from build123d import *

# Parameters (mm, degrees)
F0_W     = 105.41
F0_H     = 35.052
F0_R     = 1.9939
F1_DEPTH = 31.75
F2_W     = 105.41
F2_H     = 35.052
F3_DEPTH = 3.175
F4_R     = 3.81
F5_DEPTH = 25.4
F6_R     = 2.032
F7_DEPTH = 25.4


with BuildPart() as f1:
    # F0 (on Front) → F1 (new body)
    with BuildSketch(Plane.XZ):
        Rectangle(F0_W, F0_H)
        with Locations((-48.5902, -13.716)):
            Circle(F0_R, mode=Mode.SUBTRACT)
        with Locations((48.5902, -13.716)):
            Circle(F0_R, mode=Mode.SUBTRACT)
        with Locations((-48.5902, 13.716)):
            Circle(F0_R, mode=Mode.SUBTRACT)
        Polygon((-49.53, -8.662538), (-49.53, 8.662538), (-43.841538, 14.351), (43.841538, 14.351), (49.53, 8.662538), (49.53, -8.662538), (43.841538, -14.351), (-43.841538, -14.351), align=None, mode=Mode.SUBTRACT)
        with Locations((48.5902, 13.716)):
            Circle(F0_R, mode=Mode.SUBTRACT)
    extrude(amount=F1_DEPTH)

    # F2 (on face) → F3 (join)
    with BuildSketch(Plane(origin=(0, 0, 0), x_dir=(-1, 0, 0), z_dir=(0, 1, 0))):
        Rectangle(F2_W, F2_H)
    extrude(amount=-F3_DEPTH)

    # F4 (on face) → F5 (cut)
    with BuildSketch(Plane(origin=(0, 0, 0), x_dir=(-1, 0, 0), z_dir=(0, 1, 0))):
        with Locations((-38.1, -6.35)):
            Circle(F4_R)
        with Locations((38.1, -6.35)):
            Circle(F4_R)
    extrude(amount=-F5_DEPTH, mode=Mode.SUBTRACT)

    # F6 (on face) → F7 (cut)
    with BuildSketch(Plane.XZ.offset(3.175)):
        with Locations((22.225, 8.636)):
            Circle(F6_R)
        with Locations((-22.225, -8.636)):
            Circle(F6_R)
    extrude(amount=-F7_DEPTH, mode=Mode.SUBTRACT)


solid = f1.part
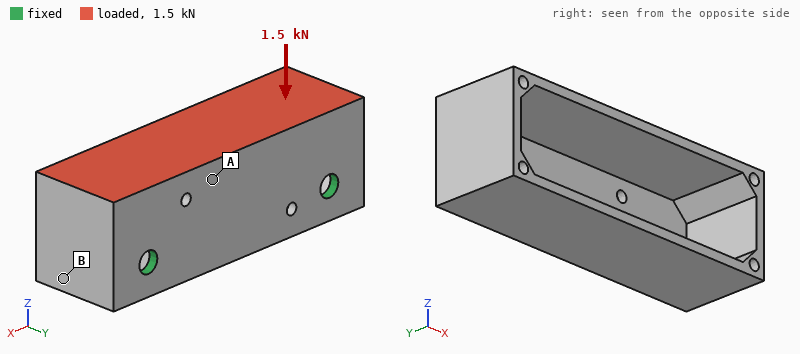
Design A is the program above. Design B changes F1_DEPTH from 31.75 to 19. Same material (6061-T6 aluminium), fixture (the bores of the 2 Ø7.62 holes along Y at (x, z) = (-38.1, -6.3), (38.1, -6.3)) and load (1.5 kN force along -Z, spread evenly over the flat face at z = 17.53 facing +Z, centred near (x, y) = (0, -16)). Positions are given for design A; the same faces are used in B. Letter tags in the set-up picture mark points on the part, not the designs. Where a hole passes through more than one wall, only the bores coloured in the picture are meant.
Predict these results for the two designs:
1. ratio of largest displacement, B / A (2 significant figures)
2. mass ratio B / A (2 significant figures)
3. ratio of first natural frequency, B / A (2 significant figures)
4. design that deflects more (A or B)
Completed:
0.45
0.69
1.5
A
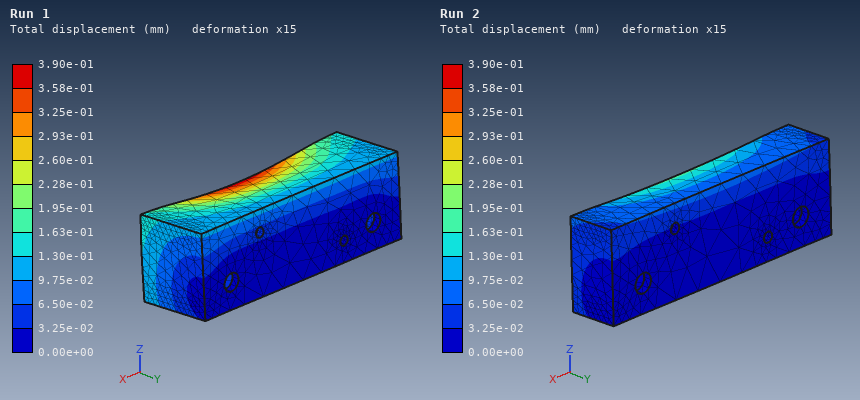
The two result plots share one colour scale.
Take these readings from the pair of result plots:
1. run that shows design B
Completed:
Run 2
